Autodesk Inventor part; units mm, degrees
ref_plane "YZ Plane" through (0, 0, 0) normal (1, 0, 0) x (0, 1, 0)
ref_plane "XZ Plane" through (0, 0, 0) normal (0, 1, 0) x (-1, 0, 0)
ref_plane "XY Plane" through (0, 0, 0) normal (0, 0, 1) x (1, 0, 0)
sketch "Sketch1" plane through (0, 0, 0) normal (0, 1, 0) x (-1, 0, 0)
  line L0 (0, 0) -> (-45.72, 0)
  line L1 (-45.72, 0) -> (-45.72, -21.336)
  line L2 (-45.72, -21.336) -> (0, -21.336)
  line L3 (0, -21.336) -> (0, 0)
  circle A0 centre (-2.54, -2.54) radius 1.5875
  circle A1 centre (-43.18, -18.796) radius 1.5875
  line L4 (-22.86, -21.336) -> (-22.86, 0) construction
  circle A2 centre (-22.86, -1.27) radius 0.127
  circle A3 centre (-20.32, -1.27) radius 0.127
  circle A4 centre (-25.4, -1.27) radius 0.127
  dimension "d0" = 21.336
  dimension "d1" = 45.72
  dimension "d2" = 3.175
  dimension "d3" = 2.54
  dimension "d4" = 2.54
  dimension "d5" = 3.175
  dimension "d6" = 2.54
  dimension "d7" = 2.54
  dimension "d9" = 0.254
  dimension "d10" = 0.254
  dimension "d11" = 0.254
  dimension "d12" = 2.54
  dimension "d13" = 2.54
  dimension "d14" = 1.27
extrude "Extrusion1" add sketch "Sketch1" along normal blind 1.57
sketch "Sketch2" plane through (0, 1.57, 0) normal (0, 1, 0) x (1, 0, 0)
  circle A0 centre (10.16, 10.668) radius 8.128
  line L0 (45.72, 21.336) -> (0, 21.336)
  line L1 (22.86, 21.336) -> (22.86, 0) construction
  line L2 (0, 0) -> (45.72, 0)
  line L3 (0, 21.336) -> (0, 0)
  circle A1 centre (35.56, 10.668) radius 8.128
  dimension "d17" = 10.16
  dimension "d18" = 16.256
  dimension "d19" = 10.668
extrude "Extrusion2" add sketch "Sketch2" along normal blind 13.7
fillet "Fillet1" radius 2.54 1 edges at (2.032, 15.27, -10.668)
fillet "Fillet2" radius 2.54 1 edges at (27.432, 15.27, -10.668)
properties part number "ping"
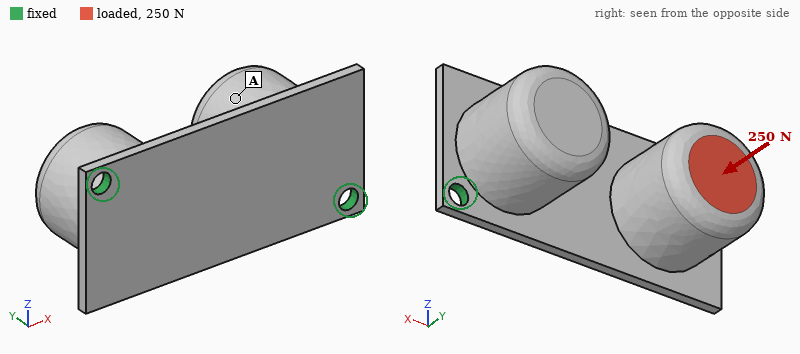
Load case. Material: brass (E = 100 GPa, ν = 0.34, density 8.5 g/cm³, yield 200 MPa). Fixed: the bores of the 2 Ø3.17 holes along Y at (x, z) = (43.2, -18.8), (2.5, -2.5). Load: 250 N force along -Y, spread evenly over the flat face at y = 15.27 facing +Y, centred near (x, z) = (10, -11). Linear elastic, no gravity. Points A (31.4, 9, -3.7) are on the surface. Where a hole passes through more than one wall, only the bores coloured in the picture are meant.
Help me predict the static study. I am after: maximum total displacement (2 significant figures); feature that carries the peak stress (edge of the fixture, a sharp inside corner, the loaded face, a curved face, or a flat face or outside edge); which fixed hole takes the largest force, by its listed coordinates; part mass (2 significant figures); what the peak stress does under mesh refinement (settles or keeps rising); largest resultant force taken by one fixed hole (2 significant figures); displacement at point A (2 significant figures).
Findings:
0.11 mm
edge of the fixture
(2.5, -2.5)
60 g
keeps rising
200 N
0.045 mm
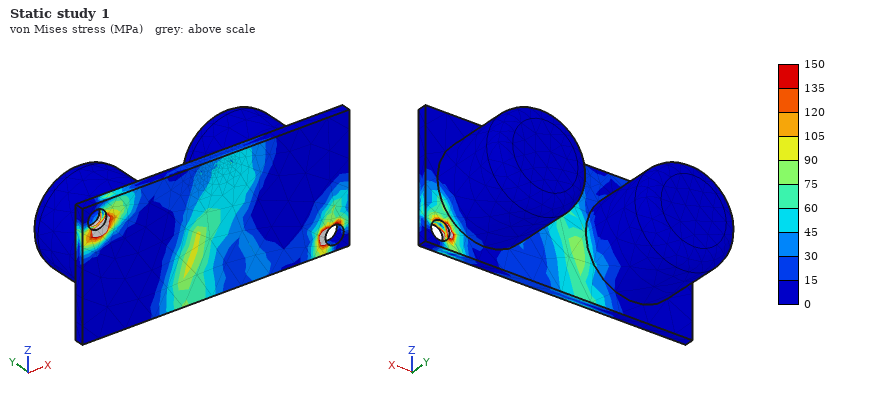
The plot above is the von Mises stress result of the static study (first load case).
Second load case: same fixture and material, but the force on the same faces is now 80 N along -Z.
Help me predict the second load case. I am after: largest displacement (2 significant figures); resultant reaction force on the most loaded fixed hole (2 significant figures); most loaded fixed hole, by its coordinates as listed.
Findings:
72 µm
70 N
(2.5, -2.5)
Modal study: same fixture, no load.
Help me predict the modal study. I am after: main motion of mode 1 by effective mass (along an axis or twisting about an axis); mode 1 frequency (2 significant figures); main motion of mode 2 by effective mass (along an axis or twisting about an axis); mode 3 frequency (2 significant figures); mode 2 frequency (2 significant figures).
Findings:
along Y
1200 Hz
along Z
2200 Hz
1400 Hz
